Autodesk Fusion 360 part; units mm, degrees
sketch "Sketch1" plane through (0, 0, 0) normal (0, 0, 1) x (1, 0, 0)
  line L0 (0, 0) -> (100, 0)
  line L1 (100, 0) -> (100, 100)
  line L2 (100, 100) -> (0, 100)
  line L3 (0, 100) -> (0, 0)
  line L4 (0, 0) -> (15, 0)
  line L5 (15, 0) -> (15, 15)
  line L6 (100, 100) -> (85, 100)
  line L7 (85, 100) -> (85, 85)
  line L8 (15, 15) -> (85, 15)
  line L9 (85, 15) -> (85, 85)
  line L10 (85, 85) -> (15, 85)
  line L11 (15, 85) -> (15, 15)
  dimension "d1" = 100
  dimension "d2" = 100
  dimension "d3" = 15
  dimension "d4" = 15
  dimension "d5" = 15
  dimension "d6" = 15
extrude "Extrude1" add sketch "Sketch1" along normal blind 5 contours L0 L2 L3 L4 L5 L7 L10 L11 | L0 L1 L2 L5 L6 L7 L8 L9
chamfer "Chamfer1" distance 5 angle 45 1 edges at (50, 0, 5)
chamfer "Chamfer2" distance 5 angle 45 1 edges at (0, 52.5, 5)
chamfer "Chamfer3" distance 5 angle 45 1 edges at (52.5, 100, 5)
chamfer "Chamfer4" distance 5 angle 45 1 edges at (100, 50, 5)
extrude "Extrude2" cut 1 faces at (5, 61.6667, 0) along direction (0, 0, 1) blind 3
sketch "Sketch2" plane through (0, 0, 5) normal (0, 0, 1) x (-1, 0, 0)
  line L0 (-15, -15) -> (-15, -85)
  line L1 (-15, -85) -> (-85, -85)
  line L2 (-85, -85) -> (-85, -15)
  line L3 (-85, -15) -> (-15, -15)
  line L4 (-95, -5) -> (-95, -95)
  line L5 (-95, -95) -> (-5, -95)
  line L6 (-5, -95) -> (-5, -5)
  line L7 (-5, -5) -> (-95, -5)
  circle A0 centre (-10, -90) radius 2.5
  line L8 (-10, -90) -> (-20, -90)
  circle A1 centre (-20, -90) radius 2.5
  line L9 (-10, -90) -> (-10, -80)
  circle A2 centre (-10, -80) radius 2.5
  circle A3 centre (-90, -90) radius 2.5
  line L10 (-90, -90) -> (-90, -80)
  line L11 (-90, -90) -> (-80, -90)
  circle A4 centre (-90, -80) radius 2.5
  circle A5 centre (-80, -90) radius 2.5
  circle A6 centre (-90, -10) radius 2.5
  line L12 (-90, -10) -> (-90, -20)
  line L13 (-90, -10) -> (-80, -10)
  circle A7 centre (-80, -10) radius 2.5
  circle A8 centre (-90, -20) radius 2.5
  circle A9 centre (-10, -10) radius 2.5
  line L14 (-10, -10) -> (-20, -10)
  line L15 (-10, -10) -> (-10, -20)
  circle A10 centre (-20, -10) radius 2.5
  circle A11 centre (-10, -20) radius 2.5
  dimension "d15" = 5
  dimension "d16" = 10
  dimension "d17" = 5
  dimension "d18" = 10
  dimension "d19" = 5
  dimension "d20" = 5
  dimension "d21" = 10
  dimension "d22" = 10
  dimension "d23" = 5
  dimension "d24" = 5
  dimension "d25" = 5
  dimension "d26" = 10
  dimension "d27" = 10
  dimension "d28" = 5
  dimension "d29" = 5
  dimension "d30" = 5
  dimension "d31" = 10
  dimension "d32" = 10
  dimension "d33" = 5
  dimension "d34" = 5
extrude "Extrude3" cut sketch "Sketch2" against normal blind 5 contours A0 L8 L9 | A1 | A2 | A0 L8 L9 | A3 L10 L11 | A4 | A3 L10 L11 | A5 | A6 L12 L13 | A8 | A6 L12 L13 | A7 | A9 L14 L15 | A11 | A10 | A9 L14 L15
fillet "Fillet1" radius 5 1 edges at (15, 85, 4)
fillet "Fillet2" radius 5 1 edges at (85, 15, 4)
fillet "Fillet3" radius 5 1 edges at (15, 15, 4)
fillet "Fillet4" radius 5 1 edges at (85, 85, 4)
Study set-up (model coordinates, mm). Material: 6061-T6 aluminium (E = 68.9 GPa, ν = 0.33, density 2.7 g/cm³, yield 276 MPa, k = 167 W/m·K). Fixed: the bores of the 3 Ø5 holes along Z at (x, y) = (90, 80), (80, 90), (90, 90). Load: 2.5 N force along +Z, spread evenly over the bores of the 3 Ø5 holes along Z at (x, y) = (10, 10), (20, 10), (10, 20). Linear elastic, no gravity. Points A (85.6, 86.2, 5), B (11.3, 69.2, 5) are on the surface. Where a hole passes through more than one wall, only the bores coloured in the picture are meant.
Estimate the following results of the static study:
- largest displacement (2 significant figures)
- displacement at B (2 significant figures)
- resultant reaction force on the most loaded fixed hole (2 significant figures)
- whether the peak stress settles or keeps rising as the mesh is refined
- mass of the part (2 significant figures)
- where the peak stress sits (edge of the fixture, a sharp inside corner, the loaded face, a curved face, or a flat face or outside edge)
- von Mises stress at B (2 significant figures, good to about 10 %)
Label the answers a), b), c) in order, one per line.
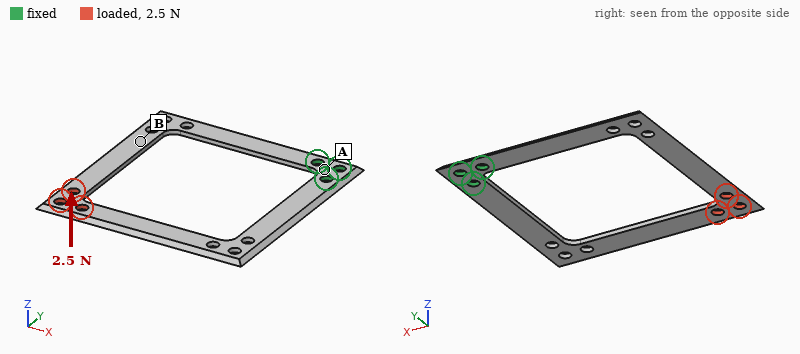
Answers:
a) 1.4 mm
b) 0.53 mm
c) 1.7 N
d) keeps rising
e) 18 g
f) edge of the fixture
g) 6.9 MPa
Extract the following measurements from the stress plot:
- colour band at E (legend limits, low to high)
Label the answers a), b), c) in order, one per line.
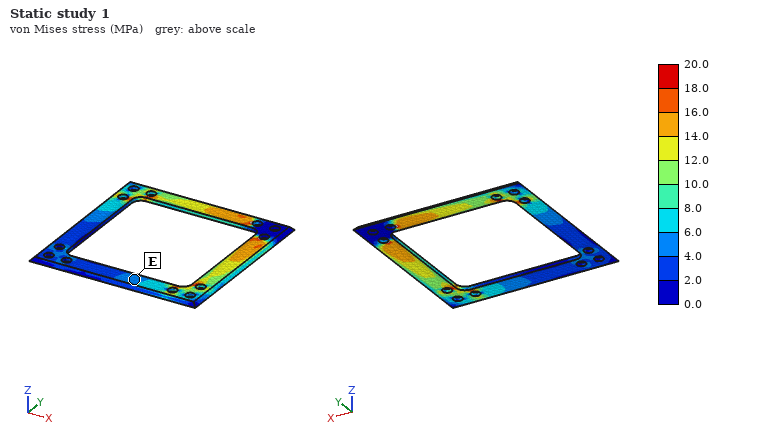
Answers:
a) 4.0 to 6.0 MPa
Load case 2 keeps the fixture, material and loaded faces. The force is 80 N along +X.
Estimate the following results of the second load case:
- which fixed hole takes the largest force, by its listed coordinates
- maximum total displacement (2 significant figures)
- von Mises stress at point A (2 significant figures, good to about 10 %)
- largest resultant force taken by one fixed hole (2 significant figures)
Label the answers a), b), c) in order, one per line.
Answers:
a) (90, 80)
b) 0.40 mm
c) 7.5 MPa
d) 150 N
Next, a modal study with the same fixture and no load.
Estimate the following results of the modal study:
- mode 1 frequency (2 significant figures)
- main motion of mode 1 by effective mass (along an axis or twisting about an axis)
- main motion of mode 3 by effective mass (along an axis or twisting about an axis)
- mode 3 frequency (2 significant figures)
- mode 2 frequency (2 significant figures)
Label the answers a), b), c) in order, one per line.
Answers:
a) 110 Hz
b) along Z
c) along Z
d) 430 Hz
e) 230 Hz
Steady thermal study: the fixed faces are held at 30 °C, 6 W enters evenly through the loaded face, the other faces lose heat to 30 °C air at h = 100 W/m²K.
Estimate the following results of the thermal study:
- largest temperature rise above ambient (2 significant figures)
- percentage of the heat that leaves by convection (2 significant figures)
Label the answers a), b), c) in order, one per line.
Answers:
a) 28 K
b) 96 %
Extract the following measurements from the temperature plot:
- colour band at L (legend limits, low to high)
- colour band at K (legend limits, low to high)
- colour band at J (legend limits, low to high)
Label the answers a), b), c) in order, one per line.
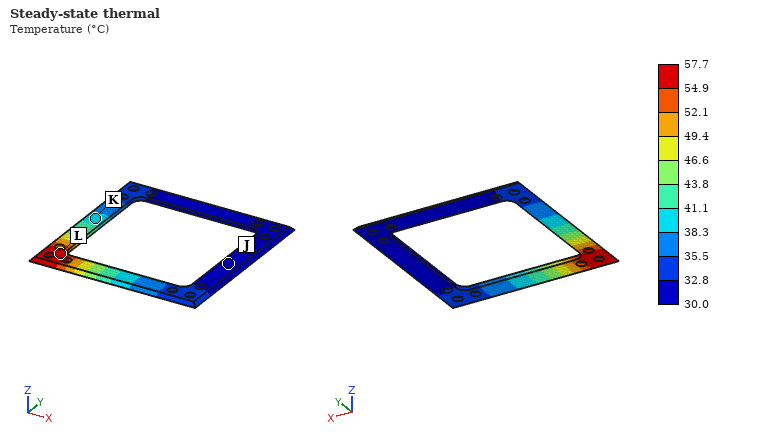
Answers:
a) 54.9 to 57.7 °C
b) 38.3 to 41.1 °C
c) 30.0 to 32.8 °C
